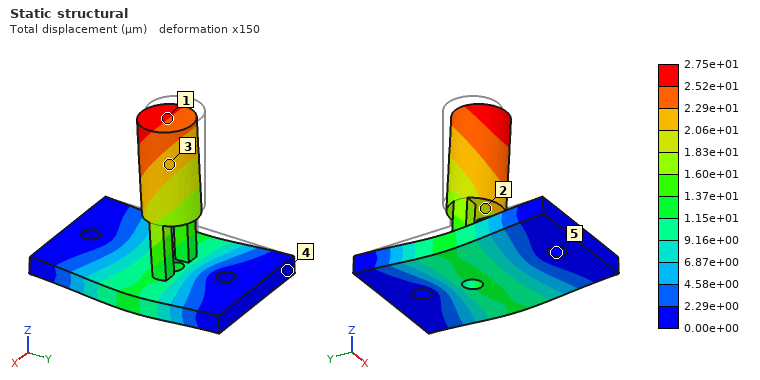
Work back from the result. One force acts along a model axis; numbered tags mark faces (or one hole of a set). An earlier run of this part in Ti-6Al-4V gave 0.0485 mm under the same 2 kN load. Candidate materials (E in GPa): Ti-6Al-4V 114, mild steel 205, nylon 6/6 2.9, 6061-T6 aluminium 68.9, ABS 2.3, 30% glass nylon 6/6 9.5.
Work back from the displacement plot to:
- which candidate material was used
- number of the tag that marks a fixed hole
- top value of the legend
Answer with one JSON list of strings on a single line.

["mild steel", "5", "2.75e+01 µm"]
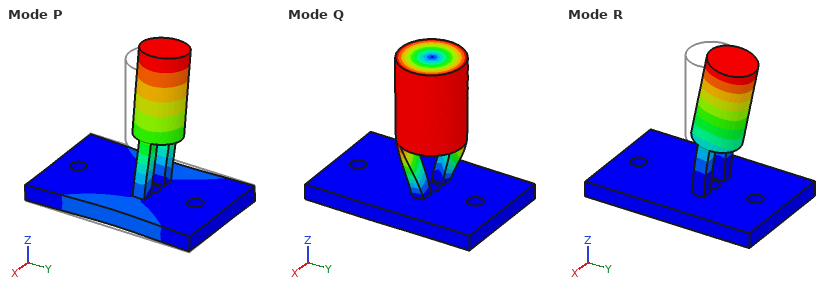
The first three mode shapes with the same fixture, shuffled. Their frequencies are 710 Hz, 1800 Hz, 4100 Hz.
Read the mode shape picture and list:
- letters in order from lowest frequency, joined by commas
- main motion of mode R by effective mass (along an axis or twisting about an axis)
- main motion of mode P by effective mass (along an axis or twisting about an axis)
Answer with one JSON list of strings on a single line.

["R, P, Q", "along Y", "along X"]
